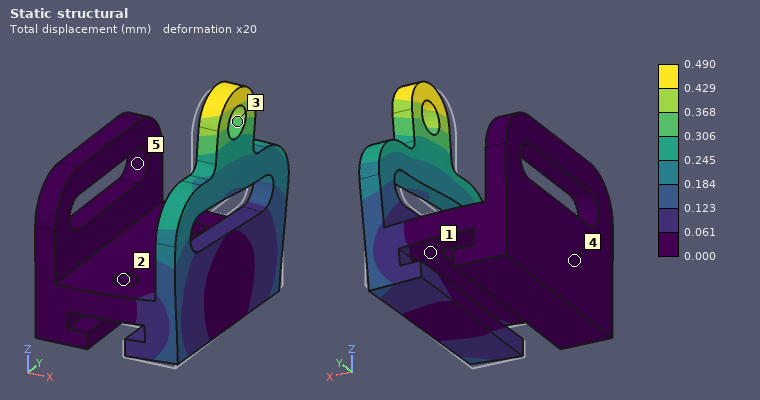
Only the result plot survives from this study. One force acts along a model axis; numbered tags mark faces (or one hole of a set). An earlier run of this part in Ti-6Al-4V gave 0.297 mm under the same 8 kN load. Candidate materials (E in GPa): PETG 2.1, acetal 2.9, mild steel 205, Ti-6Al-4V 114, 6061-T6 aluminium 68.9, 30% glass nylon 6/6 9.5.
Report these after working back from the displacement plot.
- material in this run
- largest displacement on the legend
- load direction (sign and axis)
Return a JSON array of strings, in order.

["6061-T6 aluminium", "0.490 mm", "+Y"]
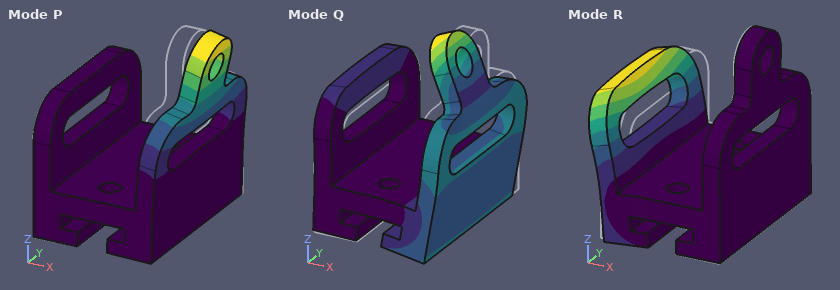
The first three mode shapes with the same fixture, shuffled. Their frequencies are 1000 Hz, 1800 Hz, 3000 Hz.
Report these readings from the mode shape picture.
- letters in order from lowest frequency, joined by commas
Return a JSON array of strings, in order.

["P, R, Q"]
